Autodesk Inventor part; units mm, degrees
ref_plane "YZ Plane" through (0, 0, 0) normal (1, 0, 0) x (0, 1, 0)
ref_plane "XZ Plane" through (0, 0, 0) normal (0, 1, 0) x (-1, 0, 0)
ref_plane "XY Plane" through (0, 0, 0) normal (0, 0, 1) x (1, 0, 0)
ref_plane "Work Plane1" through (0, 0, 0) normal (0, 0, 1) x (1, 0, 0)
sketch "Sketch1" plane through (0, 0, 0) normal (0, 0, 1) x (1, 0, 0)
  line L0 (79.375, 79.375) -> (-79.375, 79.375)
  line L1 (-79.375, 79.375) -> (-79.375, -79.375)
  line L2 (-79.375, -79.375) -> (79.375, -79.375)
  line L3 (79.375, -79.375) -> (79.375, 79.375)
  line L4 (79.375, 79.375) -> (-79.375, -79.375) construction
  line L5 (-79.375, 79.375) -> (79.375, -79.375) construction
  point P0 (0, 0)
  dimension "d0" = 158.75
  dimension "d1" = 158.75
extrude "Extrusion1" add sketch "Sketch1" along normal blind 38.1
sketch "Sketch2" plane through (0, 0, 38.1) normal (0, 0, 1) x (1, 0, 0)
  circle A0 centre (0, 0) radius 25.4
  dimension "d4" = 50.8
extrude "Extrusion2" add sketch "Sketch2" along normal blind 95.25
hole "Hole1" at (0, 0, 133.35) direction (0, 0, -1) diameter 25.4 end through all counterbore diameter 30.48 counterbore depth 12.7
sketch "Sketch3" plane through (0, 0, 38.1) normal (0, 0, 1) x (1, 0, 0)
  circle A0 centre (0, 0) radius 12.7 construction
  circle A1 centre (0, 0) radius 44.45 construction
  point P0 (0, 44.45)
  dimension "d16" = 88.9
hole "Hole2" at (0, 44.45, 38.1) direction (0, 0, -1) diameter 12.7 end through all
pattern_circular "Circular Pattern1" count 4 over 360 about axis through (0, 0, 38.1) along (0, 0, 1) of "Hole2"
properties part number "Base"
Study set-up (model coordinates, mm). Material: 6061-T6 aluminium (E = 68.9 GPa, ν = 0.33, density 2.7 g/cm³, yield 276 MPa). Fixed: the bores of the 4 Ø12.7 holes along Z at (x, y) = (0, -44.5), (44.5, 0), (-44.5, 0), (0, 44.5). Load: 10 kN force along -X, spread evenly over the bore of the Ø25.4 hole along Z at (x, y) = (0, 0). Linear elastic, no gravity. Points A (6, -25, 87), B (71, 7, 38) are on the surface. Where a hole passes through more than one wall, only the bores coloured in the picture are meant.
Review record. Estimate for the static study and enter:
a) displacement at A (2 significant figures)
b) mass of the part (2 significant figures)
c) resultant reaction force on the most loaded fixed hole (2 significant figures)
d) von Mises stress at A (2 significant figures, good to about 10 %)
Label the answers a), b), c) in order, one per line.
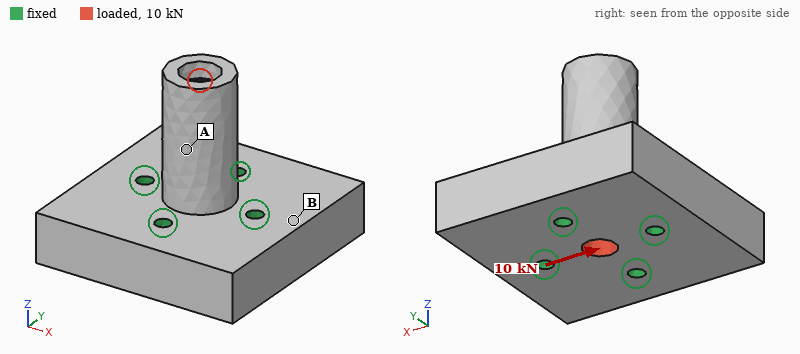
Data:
a) 29 µm
b) 2.9 kg
c) 5.6 kN
d) 4.9 MPa
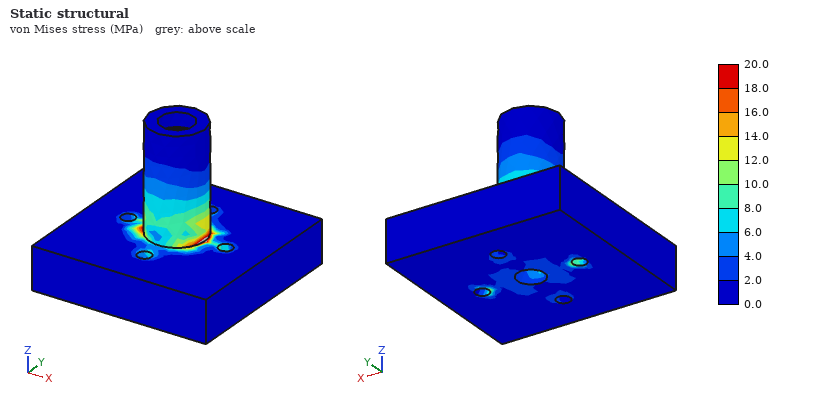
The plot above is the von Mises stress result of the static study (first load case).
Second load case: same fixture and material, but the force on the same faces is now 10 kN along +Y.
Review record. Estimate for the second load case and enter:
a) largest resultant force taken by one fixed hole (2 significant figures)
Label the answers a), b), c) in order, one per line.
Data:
a) 5.6 kN
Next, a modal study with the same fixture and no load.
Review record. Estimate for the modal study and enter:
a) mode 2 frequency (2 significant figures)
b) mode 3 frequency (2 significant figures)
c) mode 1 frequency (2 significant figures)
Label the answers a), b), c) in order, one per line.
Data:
a) 3100 Hz
b) 6000 Hz
c) 3100 Hz
